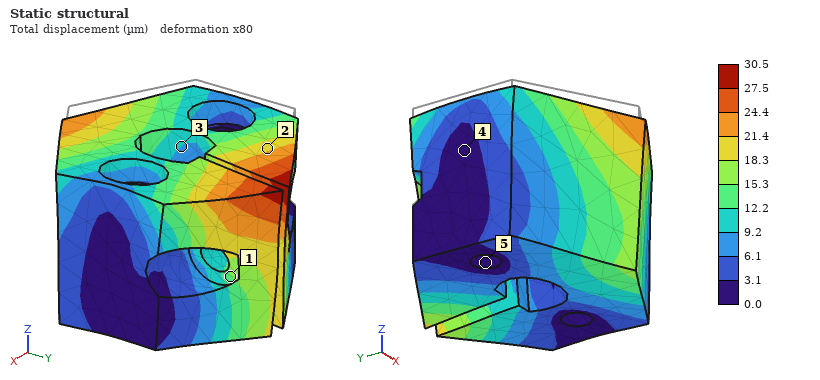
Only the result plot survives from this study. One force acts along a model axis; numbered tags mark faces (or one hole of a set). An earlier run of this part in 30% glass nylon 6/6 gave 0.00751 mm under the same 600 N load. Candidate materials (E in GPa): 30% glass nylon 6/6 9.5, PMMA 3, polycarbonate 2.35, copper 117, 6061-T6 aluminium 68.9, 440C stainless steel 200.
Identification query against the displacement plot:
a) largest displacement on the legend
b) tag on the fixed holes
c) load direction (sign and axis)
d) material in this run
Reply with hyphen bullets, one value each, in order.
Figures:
- 30.5 µm
- 5
- -Z
- polycarbonate
